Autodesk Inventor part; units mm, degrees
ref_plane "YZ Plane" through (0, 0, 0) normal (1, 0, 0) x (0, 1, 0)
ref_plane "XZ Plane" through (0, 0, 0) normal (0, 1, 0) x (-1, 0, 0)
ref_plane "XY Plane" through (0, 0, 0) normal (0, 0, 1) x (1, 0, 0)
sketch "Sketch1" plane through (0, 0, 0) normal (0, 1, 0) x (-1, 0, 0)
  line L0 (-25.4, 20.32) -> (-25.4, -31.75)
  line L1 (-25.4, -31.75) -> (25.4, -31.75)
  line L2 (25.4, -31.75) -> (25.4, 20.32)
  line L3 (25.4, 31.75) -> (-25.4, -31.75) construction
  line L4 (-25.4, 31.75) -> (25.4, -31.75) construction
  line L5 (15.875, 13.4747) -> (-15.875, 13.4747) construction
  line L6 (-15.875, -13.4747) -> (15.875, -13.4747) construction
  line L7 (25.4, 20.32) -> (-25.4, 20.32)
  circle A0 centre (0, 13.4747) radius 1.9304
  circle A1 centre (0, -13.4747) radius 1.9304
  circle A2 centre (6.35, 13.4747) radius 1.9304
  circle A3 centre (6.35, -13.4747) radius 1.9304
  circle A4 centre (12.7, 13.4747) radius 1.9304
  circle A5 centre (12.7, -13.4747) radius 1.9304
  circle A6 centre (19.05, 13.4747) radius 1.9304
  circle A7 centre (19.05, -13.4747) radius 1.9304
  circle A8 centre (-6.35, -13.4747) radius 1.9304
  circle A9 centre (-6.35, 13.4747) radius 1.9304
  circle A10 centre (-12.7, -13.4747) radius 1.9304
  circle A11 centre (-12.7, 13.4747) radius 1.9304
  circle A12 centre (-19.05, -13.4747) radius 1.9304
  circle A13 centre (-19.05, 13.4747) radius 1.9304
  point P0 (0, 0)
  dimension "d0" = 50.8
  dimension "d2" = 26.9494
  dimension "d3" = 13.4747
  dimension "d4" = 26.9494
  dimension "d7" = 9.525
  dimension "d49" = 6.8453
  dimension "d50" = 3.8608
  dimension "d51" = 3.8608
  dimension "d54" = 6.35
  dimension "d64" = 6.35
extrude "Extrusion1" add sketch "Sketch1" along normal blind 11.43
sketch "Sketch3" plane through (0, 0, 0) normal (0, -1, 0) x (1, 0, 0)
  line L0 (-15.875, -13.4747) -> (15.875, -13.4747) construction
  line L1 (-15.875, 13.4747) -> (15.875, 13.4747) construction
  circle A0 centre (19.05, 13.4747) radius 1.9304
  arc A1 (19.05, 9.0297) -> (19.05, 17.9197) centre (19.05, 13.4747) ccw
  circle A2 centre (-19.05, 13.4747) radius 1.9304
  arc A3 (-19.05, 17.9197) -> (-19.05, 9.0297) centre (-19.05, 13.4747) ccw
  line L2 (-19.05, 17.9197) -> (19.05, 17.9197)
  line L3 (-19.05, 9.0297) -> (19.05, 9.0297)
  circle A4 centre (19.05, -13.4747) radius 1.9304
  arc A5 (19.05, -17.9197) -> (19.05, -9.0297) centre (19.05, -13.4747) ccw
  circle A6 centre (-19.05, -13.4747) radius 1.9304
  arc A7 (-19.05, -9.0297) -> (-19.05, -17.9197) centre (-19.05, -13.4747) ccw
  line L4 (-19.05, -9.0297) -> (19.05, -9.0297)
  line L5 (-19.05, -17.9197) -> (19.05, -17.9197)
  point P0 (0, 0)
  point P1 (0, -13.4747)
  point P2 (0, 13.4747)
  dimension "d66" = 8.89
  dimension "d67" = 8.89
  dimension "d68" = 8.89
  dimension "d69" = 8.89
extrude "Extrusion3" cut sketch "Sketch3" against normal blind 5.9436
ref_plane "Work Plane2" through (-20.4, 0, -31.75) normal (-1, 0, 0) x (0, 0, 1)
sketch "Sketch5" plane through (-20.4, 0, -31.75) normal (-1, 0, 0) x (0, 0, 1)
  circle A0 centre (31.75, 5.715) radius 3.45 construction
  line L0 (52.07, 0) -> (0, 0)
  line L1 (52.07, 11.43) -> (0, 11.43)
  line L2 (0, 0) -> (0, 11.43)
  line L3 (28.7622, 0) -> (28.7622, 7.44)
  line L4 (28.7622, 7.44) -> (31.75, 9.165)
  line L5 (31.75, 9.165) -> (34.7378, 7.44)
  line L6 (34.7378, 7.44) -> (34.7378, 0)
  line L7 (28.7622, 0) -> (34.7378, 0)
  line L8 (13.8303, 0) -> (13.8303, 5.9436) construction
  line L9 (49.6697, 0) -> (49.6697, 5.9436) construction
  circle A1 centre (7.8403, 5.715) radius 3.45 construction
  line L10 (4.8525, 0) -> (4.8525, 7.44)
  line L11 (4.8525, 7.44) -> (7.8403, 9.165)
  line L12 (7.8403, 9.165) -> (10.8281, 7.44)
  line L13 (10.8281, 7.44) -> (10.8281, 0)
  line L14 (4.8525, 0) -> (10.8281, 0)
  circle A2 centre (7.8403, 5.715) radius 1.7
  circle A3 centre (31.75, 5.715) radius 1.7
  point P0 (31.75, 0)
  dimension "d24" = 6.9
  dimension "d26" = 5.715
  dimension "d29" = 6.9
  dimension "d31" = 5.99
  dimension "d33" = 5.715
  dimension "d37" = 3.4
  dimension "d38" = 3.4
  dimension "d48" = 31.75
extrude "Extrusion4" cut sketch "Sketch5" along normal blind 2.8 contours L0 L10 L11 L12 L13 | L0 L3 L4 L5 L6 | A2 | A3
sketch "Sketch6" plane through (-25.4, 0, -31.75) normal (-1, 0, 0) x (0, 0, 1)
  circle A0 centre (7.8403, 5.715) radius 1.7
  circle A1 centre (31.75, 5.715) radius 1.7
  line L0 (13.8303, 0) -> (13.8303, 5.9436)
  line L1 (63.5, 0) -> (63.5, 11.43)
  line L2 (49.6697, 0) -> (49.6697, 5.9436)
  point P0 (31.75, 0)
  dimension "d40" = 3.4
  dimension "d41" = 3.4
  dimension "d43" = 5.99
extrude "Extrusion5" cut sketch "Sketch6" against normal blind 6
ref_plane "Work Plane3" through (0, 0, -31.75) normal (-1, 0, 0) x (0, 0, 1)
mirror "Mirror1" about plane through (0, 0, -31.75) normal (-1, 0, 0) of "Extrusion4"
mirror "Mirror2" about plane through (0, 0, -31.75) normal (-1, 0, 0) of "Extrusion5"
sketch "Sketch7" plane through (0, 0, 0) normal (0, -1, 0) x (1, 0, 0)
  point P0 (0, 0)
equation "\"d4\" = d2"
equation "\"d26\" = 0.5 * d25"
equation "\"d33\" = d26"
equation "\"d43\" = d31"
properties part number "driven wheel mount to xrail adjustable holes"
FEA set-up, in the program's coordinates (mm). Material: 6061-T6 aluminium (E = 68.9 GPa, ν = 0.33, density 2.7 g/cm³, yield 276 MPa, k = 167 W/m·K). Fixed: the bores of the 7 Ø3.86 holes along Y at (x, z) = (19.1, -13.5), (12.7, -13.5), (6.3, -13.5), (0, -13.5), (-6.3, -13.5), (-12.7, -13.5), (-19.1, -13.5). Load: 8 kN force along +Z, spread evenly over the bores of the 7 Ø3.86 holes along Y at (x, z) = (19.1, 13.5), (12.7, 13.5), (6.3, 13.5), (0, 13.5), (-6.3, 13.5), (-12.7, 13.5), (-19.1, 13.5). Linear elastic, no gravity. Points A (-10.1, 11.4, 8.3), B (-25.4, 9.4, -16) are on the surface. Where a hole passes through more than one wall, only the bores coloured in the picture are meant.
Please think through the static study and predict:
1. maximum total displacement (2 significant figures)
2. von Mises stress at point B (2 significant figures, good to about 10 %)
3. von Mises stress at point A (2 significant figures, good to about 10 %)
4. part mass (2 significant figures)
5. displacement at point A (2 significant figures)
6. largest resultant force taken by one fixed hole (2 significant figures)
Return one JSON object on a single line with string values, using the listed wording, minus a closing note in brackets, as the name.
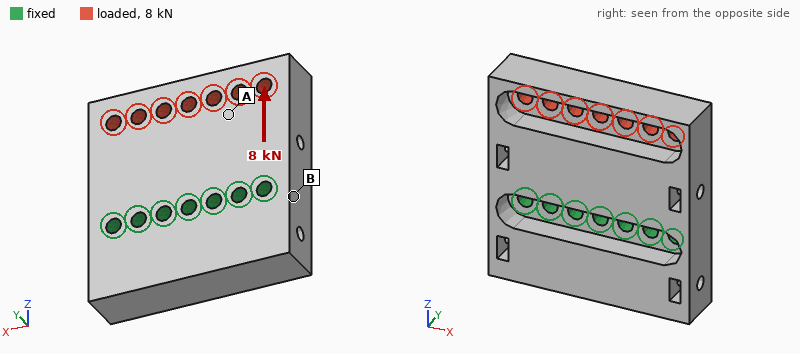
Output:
{"maximum total displacement": "24 µm", "von Mises stress at point B": "11 MPa", "von Mises stress at point A": "36 MPa", "part mass": "65 g", "displacement at point A": "14 µm", "largest resultant force taken by one fixed hole": "1.4 kN"}
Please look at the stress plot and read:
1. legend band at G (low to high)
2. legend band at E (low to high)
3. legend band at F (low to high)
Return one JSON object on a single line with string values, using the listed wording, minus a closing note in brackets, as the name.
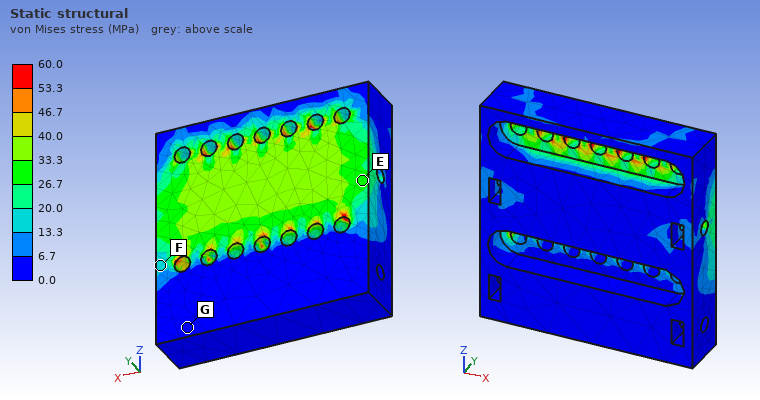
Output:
{"legend band at G": "0.0 to 6.7 MPa", "legend band at E": "26.7 to 33.3 MPa", "legend band at F": "13.3 to 20.0 MPa"}
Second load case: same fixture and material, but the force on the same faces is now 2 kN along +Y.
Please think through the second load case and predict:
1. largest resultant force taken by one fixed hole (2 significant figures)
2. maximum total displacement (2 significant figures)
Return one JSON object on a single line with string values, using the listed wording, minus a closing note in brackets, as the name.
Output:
{"largest resultant force taken by one fixed hole": "420 N", "maximum total displacement": "0.16 mm"}
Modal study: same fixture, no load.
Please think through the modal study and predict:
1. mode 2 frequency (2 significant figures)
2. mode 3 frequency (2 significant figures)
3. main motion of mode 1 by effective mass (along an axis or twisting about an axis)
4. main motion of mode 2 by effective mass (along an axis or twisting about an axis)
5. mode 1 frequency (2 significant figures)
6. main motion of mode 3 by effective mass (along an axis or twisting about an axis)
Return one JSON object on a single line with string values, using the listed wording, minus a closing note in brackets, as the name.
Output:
{"mode 2 frequency": "9300 Hz", "mode 3 frequency": "12 kHz", "main motion of mode 1 by effective mass": "along Y", "main motion of mode 2 by effective mass": "twisting about Z", "mode 1 frequency": "4900 Hz", "main motion of mode 3 by effective mass": "along Y"}
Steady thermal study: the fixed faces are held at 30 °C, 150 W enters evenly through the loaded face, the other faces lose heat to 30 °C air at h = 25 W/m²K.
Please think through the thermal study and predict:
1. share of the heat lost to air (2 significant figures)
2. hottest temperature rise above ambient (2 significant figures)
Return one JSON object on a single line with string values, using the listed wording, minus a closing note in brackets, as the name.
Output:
{"share of the heat lost to air": "3.7 %", "hottest temperature rise above ambient": "71 K"}
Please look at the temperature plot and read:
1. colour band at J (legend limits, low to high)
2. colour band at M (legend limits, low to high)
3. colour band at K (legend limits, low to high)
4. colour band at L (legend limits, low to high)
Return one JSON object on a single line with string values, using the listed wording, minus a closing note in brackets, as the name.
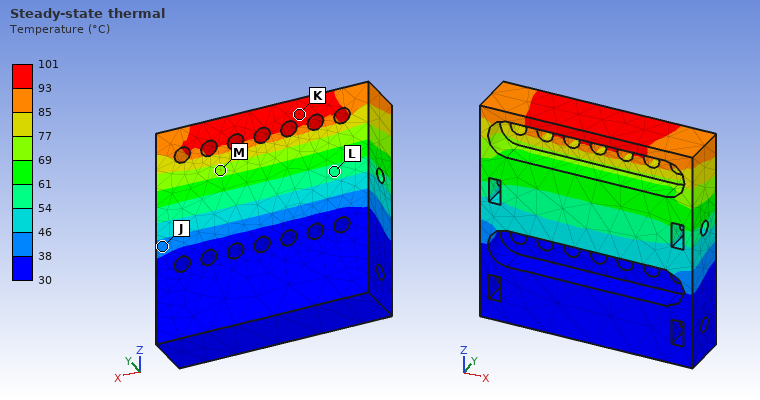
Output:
{"colour band at J": "38 to 46 °C", "colour band at M": "69 to 77 °C", "colour band at K": "93 to 101 °C", "colour band at L": "54 to 61 °C"}
